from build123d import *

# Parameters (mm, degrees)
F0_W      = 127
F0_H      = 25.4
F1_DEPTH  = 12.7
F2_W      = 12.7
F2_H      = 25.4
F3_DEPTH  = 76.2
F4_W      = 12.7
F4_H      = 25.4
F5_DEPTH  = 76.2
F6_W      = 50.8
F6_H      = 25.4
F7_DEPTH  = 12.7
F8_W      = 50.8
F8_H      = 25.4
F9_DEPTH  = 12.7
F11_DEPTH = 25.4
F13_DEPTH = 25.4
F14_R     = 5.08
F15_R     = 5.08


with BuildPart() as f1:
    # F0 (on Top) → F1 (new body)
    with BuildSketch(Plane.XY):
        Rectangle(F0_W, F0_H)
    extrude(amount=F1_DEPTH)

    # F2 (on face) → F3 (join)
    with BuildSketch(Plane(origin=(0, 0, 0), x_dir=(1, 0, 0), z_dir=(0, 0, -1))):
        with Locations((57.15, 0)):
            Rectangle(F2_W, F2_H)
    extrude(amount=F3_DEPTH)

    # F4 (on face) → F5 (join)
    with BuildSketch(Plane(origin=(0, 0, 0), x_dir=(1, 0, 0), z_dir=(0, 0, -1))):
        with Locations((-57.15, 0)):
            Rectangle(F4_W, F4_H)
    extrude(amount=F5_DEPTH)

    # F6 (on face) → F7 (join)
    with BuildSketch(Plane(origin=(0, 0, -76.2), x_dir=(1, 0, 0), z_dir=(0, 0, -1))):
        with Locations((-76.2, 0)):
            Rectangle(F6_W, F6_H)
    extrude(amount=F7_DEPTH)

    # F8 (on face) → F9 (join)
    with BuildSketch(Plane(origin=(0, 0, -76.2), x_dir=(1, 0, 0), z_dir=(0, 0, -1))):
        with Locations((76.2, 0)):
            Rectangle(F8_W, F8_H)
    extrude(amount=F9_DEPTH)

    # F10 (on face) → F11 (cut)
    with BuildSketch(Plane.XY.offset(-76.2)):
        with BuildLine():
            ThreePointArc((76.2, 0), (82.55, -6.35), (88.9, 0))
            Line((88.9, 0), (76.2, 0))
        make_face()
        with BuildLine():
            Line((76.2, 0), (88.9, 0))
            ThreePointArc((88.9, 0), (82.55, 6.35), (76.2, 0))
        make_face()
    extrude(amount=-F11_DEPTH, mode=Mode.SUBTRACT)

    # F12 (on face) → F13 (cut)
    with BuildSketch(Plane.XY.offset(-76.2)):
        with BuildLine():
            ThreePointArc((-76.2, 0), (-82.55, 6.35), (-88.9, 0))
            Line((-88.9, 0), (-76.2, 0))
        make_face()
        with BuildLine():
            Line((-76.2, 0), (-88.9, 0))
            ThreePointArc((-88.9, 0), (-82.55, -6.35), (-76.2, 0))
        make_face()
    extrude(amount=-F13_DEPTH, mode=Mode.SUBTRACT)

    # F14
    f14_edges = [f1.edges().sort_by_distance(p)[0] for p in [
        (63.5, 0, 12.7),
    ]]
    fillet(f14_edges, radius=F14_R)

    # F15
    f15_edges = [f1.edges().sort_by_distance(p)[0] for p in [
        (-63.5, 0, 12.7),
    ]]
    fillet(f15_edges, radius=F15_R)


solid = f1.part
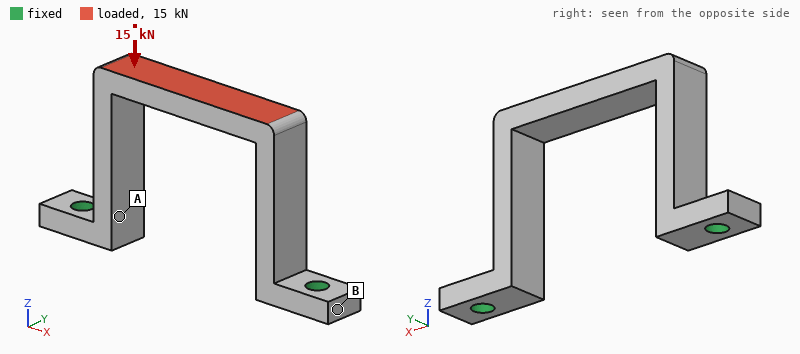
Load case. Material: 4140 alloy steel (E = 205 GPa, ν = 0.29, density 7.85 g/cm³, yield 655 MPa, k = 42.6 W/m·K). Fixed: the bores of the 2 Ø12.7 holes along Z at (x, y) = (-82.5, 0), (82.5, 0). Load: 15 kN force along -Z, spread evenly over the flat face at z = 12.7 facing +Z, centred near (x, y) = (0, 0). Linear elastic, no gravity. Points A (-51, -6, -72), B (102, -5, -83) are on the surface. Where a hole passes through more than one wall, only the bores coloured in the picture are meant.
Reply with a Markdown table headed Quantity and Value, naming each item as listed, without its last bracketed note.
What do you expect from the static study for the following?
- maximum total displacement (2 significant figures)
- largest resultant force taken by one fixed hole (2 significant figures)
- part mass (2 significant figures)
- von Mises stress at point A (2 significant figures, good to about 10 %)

| Quantity | Value |
|---|---|
| maximum total displacement | 0.15 mm |
| largest resultant force taken by one fixed hole | 7.8 kN |
| part mass | 940 g |
| von Mises stress at point A | 45 MPa |
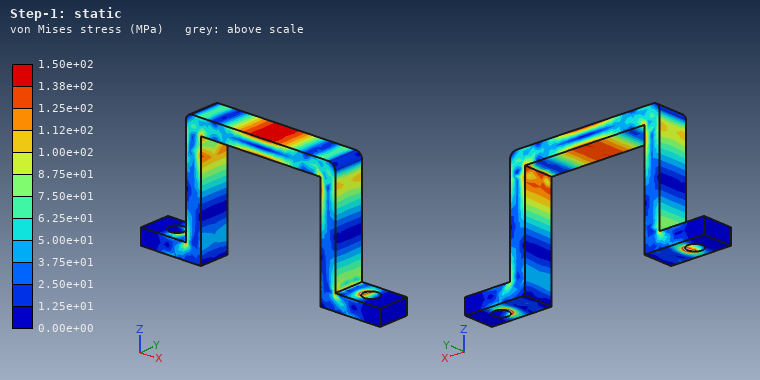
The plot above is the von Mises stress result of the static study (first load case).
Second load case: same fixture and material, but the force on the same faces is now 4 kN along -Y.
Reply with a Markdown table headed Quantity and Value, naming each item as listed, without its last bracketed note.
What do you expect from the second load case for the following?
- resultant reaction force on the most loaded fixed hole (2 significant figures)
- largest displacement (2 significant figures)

| Quantity | Value |
|---|---|
| resultant reaction force on the most loaded fixed hole | 2.0 kN |
| largest displacement | 0.49 mm |
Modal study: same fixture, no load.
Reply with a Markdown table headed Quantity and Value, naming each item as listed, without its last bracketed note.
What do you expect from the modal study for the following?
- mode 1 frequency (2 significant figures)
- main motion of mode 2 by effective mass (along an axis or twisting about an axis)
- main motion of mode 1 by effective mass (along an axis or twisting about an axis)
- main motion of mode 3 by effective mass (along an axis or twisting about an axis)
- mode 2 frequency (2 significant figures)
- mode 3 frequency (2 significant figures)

| Quantity | Value |
|---|---|
| mode 1 frequency | 770 Hz |
| main motion of mode 2 by effective mass | along X |
| main motion of mode 1 by effective mass | along Y |
| main motion of mode 3 by effective mass | twisting about Z |
| mode 2 frequency | 950 Hz |
| mode 3 frequency | 1500 Hz |
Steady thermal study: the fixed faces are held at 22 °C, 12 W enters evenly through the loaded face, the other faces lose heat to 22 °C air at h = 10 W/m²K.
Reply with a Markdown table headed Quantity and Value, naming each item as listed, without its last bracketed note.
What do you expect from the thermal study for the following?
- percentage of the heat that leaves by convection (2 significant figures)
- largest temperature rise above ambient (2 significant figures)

| Quantity | Value |
|---|---|
| percentage of the heat that leaves by convection | 37 % |
| largest temperature rise above ambient | 40 K |
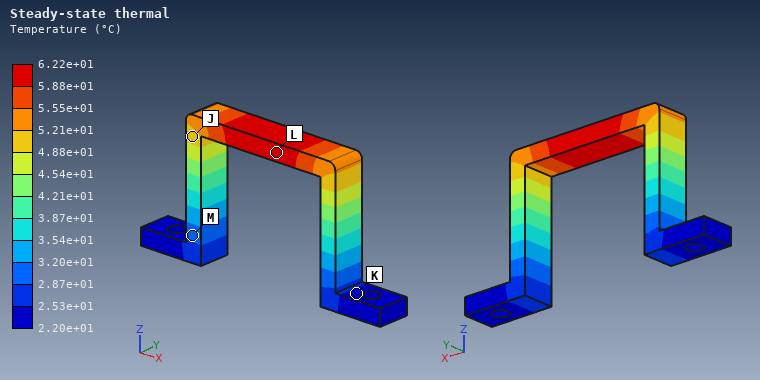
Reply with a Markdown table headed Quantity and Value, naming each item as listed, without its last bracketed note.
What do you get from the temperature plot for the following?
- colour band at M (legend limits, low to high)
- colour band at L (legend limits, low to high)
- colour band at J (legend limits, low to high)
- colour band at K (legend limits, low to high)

| Quantity | Value |
|---|---|
| colour band at M | 2.87e+01 to 3.20e+01 °C |
| colour band at L | 5.88e+01 to 6.22e+01 °C |
| colour band at J | 4.88e+01 to 5.21e+01 °C |
| colour band at K | 2.20e+01 to 2.53e+01 °C |
